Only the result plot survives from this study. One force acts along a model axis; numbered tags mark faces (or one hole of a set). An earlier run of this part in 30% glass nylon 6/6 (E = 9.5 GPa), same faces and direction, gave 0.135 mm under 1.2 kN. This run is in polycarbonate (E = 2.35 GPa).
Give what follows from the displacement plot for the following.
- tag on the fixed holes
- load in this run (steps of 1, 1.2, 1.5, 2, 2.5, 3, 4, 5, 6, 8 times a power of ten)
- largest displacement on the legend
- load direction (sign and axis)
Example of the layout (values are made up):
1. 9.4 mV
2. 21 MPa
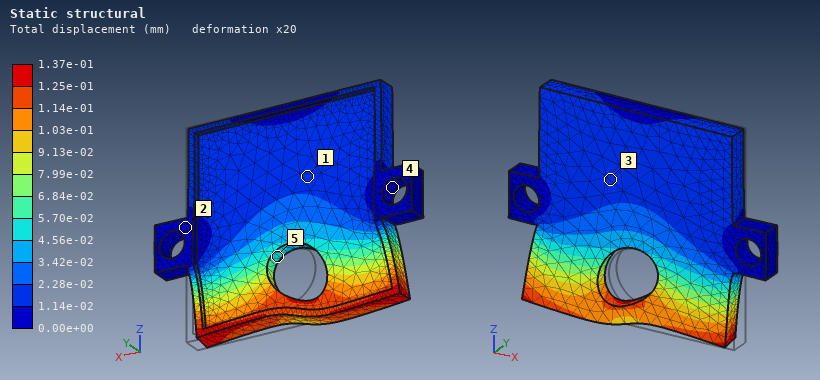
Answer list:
1. 4
2. 300 N
3. 1.37e-01 mm
4. -X
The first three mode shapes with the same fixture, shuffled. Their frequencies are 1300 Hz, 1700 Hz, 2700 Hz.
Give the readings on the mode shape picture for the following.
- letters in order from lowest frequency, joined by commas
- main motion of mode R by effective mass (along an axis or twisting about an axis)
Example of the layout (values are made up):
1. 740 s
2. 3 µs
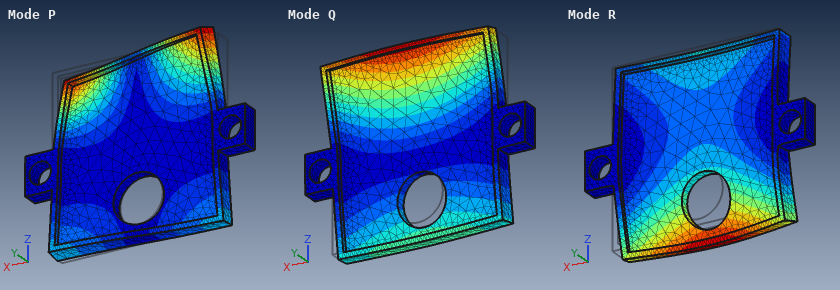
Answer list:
1. Q, R, P
2. along Y
